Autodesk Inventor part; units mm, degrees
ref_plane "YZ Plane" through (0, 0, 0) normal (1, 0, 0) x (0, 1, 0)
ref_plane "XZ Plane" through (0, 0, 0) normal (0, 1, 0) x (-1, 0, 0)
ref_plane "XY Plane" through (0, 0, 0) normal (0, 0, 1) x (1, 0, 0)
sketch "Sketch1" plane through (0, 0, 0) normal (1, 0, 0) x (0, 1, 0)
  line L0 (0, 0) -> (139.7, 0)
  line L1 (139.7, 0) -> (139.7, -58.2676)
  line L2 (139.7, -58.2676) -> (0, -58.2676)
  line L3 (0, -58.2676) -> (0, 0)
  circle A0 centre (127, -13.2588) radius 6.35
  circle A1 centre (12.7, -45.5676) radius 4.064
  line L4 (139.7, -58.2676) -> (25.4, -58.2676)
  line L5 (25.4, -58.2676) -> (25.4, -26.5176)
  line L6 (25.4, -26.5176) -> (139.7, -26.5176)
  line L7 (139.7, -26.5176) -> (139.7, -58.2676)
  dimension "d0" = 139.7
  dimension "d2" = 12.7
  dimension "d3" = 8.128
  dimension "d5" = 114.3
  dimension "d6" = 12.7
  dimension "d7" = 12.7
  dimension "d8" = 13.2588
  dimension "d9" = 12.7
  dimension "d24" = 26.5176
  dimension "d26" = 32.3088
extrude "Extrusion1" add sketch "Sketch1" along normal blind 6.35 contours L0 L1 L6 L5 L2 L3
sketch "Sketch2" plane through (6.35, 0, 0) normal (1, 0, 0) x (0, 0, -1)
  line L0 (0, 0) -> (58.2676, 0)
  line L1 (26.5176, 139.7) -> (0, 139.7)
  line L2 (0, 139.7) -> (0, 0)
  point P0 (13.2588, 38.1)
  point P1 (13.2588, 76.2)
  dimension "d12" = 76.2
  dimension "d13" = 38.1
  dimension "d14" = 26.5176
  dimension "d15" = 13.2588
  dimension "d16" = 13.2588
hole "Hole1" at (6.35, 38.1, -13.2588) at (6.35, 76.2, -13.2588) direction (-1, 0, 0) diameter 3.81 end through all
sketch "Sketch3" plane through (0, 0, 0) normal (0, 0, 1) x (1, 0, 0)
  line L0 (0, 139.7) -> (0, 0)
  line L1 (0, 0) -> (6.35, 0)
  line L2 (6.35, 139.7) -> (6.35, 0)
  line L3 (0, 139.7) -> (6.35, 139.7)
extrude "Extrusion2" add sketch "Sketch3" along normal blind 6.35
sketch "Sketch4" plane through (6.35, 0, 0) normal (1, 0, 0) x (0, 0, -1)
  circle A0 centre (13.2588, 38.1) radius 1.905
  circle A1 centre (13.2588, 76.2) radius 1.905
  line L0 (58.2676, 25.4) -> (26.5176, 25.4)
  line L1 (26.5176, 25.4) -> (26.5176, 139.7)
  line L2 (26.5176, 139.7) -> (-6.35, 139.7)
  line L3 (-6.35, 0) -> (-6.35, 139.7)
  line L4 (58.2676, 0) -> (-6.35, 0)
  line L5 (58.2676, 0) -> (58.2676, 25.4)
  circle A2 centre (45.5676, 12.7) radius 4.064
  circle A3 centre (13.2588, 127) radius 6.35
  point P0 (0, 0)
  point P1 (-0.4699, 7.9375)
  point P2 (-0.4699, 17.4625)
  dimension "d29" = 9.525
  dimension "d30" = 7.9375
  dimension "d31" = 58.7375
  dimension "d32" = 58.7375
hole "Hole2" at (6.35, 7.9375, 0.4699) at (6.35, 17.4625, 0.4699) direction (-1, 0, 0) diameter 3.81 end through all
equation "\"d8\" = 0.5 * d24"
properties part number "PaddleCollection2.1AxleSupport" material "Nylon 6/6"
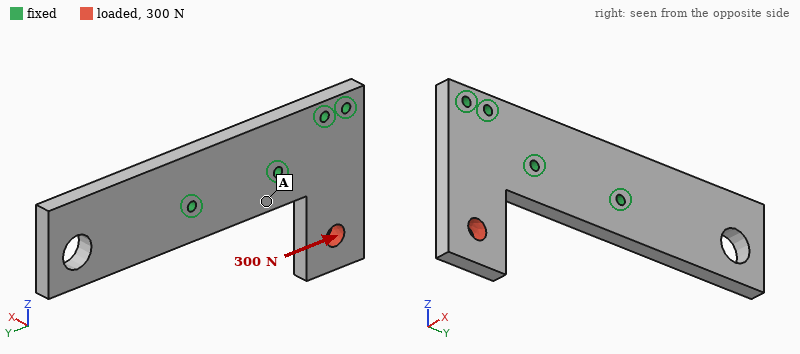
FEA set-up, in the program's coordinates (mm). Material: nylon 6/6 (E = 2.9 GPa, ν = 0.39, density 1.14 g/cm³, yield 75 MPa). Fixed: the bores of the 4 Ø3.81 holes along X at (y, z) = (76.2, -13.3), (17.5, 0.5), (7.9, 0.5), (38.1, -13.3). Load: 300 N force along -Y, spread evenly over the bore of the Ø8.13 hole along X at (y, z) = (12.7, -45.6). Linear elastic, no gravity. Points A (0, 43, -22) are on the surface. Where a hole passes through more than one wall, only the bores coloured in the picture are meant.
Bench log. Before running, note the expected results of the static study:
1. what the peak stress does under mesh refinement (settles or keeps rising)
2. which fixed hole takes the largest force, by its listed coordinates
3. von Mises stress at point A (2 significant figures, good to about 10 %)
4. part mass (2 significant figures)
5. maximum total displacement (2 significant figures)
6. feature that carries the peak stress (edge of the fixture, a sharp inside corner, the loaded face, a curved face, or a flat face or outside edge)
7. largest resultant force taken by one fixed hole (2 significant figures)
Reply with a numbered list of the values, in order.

1. keeps rising
2. (38.1, -13.3)
3. 1.4 MPa
4. 37 g
5. 0.29 mm
6. a sharp inside corner
7. 370 N
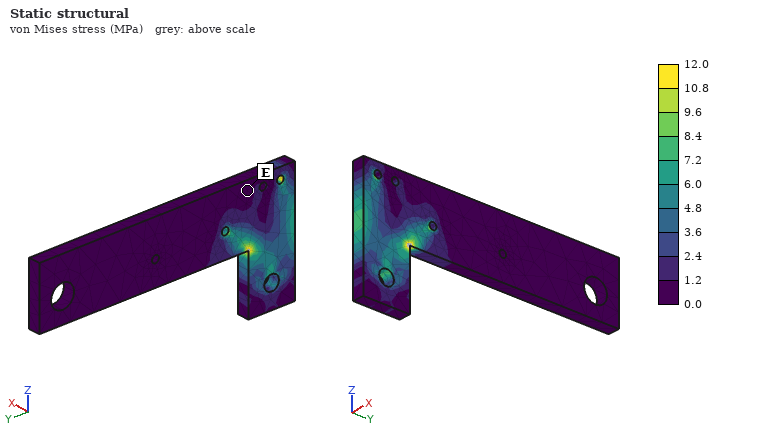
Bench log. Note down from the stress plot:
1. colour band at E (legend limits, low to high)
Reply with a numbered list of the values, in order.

1. 0.0 to 1.2 MPa
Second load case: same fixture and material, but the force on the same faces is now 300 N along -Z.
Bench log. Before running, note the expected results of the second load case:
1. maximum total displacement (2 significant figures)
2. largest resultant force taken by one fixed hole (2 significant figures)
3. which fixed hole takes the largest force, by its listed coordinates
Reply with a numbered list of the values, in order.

1. 44 µm
2. 170 N
3. (7.9, 0.5)
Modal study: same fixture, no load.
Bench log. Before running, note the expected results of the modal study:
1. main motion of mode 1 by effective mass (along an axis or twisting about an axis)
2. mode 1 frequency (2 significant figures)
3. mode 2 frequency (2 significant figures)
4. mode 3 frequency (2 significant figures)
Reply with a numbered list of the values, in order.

1. along X
2. 410 Hz
3. 660 Hz
4. 1300 Hz
